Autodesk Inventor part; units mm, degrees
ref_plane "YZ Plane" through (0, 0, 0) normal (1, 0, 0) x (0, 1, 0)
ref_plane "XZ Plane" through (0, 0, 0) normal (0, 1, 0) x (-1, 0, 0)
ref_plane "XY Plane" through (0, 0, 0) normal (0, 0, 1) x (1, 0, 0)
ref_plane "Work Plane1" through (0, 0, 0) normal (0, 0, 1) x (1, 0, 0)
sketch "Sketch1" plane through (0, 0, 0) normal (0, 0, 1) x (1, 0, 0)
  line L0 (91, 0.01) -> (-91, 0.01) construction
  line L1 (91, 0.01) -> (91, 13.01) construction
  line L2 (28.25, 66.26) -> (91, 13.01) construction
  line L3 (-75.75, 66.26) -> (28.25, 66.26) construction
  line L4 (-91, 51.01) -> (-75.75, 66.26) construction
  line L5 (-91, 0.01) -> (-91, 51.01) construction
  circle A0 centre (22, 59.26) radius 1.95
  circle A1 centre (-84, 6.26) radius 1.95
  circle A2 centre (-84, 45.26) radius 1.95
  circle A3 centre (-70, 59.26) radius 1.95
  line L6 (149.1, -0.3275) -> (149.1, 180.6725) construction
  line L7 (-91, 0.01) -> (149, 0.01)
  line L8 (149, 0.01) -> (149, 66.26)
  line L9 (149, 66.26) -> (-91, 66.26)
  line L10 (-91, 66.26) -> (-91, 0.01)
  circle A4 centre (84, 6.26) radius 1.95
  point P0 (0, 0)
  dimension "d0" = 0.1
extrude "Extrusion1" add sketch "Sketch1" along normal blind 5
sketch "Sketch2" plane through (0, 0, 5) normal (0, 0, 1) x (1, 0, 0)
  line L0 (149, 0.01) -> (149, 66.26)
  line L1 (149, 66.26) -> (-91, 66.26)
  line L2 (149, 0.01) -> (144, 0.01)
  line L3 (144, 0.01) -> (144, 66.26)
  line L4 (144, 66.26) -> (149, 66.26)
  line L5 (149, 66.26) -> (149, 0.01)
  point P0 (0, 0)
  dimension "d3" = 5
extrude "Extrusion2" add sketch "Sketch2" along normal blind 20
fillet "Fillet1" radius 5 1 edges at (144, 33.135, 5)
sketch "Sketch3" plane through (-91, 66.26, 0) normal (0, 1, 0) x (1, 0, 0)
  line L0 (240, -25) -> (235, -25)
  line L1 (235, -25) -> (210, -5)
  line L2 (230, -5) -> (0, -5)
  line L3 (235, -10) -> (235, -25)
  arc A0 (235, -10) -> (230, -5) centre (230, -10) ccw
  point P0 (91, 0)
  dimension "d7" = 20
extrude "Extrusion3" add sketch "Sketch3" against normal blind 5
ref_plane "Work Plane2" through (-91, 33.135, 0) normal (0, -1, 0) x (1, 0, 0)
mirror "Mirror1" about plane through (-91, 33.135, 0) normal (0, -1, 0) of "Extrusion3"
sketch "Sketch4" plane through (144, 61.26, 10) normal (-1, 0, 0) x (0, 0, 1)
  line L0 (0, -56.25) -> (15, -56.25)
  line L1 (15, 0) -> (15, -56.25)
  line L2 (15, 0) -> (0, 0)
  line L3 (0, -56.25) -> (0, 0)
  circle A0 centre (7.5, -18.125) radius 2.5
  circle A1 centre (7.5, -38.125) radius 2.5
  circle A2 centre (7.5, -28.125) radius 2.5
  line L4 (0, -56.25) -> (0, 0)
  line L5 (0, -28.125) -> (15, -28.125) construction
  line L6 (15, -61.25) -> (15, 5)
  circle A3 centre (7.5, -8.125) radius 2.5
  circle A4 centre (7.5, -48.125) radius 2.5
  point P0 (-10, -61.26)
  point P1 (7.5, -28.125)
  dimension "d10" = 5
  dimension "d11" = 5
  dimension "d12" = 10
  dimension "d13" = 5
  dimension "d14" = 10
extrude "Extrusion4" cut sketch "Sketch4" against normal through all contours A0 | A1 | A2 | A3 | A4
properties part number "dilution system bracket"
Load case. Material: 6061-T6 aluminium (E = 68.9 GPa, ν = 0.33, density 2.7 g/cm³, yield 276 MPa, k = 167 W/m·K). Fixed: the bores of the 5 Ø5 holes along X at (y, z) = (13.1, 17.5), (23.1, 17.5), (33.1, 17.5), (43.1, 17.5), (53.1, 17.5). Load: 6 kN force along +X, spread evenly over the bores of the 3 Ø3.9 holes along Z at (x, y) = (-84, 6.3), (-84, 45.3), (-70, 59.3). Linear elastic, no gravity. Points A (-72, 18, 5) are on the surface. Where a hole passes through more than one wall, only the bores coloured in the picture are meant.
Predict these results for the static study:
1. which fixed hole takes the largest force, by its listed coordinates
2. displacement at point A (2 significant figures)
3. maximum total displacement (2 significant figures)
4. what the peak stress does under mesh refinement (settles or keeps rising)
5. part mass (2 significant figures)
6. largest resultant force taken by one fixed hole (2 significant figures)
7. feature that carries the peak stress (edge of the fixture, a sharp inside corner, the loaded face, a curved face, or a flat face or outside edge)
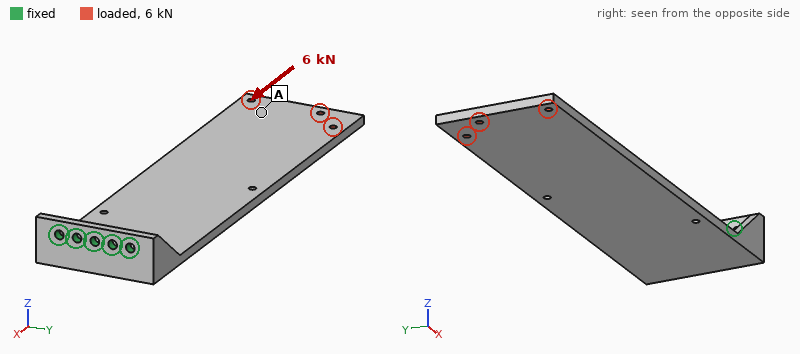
(53.1, 17.5)
1.7 mm
1.9 mm
keeps rising
240 g
1.7 kN
edge of the fixture
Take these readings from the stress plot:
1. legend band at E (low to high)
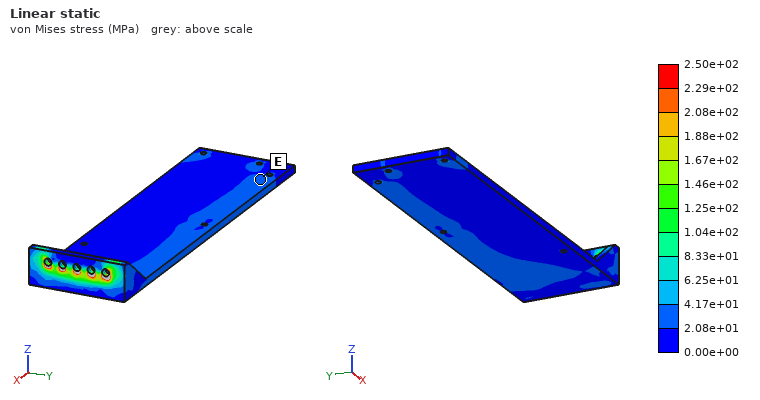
2.08e+01 to 4.17e+01 MPa
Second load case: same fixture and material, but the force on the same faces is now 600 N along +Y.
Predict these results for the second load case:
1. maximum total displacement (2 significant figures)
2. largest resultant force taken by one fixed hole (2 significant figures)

1.2 mm
2.6 kN
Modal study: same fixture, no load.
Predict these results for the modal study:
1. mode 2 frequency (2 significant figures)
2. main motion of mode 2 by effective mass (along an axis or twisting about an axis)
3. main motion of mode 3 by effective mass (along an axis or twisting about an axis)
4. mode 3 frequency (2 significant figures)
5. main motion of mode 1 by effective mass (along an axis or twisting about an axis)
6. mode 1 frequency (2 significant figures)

410 Hz
along Y
along Z
480 Hz
along Z
78 Hz
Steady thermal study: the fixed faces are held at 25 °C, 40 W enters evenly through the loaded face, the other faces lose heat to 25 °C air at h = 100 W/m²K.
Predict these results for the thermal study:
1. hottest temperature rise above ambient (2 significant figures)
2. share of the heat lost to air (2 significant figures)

41 K
96 %
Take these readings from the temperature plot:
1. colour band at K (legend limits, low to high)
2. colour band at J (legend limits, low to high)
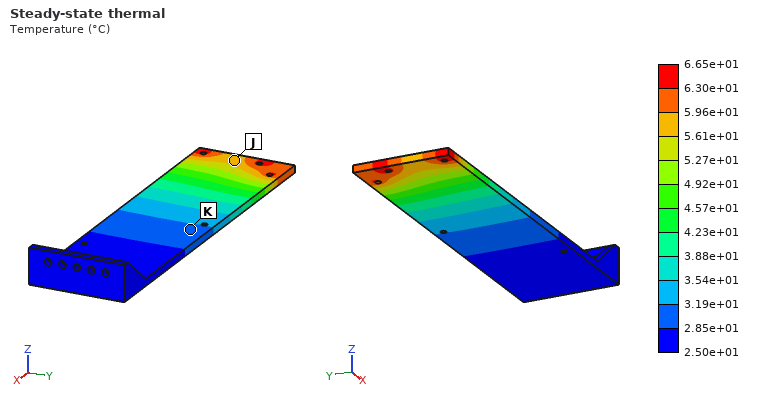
2.85e+01 to 3.19e+01 °C
5.61e+01 to 5.96e+01 °C
